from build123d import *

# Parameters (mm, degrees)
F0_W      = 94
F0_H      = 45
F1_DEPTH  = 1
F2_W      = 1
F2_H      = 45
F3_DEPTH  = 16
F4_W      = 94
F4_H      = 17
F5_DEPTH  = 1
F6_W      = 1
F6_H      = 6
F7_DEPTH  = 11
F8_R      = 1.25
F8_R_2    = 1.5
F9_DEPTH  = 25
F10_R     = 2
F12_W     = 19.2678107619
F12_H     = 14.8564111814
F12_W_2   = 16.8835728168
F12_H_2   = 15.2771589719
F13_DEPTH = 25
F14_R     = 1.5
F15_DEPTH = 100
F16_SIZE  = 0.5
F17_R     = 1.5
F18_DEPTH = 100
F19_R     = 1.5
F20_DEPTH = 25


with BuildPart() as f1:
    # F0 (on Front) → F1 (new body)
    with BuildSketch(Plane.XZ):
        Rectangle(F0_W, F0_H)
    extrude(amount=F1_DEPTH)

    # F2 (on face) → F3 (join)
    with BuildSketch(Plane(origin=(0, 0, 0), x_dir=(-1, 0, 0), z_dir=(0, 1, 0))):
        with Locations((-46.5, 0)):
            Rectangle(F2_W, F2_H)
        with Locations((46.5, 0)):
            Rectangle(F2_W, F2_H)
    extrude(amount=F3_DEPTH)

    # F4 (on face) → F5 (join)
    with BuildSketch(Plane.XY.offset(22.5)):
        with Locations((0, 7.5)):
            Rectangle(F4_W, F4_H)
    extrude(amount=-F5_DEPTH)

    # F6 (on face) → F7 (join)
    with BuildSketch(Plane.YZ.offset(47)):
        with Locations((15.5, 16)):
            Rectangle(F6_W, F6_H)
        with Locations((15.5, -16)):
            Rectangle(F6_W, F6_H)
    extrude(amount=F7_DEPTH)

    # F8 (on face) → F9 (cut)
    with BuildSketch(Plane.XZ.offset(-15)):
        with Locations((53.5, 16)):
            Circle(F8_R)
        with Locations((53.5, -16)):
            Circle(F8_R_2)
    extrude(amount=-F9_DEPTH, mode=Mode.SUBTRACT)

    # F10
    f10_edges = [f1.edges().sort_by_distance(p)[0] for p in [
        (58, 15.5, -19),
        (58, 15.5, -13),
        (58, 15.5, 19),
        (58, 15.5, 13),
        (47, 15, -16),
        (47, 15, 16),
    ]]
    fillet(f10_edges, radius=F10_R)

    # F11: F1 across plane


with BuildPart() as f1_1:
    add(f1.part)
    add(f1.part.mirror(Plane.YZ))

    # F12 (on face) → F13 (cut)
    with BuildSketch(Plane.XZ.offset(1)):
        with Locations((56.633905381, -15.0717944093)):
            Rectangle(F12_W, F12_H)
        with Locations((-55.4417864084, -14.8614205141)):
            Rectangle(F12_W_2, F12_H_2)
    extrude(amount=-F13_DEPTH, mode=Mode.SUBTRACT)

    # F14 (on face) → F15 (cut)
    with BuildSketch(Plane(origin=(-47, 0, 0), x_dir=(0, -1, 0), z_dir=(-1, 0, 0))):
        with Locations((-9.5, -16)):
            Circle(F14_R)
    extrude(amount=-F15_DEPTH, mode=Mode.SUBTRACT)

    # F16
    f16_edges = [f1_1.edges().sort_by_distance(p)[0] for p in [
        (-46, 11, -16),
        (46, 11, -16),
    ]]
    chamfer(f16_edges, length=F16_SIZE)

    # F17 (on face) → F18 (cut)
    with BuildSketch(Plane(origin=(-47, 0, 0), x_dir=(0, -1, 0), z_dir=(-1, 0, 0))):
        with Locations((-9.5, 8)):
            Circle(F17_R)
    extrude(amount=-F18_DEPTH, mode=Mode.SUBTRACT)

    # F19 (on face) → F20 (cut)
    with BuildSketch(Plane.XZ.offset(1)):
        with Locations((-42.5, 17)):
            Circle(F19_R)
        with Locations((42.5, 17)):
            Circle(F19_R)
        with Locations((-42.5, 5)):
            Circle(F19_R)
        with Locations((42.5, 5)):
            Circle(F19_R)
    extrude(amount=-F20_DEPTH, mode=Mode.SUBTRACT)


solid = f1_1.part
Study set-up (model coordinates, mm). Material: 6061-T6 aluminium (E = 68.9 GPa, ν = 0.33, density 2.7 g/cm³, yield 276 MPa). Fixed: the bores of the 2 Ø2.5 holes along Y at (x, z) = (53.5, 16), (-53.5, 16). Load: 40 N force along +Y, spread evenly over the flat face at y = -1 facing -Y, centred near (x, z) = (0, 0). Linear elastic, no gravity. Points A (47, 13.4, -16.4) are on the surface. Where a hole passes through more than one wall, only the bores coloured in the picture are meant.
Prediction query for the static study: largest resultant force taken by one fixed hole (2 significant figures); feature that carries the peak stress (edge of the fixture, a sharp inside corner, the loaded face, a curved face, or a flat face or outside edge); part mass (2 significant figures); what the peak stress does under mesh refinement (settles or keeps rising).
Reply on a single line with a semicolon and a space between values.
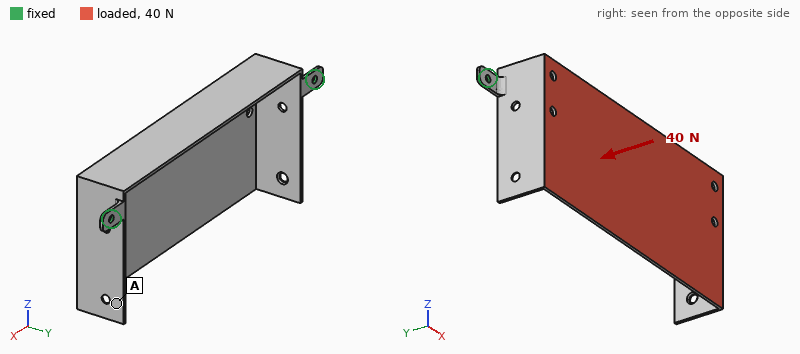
21 N; edge of the fixture; 19 g; keeps rising
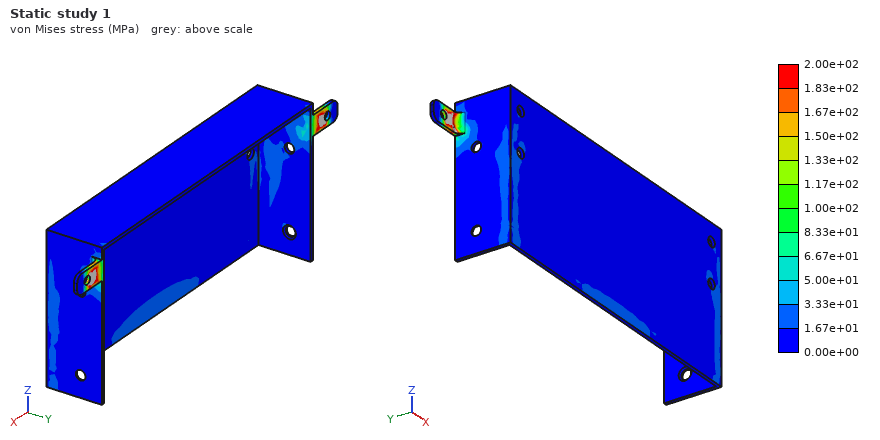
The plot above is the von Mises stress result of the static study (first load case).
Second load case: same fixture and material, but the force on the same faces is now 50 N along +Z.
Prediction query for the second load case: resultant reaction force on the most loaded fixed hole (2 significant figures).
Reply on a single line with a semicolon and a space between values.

25 N
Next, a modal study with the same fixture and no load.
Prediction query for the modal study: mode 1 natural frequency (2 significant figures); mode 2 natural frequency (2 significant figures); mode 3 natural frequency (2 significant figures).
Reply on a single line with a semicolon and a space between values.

250 Hz; 480 Hz; 750 Hz
